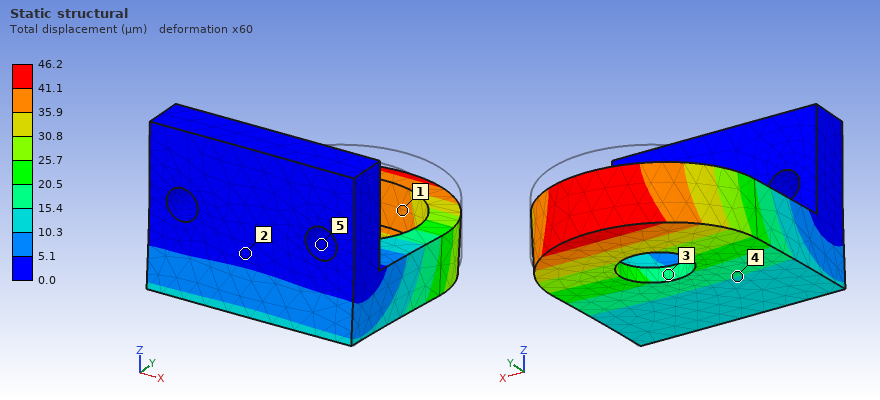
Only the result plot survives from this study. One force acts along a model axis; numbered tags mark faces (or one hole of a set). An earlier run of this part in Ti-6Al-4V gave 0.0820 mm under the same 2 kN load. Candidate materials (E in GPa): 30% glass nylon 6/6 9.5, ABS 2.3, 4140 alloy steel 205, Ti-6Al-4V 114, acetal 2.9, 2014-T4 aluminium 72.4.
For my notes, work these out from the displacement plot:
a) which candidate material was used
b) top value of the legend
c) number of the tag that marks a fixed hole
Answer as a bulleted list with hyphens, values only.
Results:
- 4140 alloy steel
- 46.2 µm
- 5
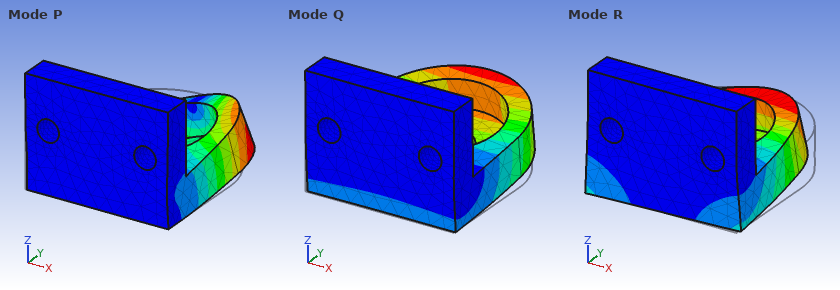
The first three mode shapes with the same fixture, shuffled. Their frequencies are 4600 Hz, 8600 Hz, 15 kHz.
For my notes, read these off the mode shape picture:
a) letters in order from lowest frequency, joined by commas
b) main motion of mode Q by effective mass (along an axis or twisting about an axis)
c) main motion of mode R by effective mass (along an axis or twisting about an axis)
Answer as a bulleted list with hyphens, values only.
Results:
- Q, R, P
- along Z
- along X
